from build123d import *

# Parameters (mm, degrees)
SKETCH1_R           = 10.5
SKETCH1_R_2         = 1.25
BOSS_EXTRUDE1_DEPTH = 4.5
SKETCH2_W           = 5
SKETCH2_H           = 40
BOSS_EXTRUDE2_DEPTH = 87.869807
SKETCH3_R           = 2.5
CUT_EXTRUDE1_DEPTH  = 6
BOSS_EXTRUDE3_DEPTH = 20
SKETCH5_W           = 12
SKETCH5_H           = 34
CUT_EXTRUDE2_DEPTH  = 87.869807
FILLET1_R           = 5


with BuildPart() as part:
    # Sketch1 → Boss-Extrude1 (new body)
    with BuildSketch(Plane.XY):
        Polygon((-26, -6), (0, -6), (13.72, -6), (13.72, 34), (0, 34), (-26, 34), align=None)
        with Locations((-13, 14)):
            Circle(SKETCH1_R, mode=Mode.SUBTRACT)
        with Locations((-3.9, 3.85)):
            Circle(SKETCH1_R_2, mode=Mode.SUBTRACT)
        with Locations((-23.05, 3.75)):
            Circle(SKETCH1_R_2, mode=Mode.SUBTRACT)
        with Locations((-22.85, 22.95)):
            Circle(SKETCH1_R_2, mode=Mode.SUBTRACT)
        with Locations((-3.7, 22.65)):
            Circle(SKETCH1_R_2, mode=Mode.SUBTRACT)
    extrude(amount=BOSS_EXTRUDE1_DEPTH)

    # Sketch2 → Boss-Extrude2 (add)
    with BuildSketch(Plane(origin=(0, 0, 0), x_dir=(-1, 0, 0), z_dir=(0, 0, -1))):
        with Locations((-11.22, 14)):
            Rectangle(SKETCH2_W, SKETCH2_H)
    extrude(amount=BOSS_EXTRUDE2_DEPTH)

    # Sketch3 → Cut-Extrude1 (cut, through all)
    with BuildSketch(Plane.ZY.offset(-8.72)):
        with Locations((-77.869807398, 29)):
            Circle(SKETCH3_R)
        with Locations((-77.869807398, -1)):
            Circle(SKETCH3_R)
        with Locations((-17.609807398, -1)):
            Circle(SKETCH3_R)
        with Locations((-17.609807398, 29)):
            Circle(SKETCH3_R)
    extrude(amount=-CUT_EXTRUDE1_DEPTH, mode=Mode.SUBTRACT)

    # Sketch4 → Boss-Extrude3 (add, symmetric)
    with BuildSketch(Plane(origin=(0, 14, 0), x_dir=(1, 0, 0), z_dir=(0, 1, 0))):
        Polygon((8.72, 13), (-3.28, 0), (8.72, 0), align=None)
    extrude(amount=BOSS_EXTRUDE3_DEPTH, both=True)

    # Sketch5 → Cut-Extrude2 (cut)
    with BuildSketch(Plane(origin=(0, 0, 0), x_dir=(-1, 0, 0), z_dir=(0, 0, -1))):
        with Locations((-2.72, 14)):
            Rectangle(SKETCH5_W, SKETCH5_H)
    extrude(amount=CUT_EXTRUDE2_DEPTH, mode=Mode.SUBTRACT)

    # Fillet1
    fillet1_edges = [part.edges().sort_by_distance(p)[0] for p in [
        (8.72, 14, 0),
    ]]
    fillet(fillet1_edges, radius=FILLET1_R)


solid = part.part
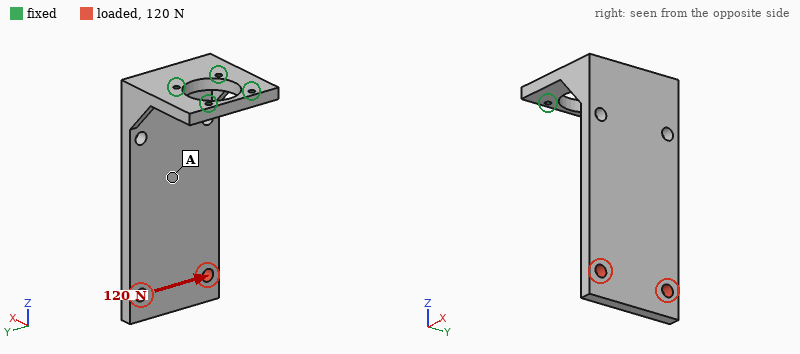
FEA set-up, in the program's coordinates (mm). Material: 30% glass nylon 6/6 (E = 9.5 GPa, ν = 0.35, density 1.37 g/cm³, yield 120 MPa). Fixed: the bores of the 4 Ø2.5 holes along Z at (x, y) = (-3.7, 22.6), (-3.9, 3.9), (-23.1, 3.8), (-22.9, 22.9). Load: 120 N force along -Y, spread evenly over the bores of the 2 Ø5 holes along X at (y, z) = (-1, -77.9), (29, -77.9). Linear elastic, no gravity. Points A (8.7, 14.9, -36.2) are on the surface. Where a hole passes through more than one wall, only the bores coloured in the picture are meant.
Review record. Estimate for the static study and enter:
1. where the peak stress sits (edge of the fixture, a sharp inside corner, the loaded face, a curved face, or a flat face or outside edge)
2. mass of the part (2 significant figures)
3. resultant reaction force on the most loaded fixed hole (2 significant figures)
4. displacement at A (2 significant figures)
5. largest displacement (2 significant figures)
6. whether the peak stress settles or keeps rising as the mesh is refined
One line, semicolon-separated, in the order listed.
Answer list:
edge of the fixture; 32 g; 400 N; 0.43 mm; 1.1 mm; keeps rising
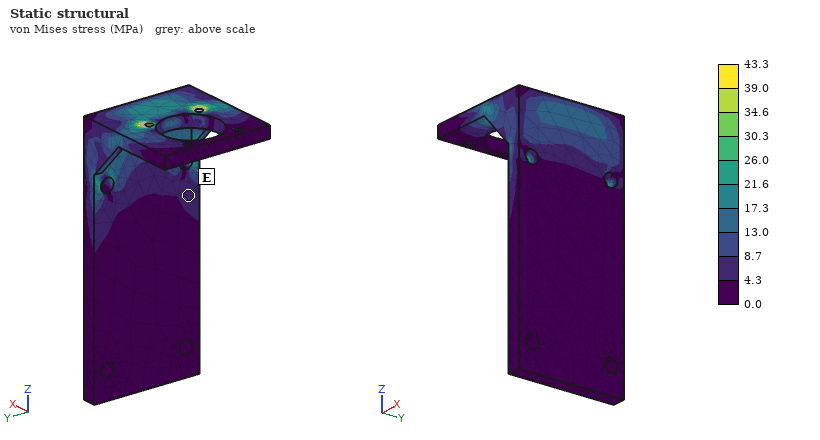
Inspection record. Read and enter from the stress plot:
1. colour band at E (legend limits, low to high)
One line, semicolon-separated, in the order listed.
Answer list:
4.3 to 8.7 MPa
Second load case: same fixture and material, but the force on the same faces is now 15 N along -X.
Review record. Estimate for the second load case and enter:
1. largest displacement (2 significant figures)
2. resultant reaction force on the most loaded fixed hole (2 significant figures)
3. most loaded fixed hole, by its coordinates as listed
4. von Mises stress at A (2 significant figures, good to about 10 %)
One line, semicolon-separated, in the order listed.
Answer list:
1.0 mm; 14 N; (-3.7, 22.6); 3.8 MPa
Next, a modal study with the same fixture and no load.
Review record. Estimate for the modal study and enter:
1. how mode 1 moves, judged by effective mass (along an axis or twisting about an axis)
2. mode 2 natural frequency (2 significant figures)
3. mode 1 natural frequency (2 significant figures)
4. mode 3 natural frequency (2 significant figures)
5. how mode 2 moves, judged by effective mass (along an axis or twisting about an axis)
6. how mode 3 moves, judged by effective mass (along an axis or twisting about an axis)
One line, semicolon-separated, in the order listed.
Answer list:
along X; 560 Hz; 220 Hz; 1200 Hz; along Y; along Z
